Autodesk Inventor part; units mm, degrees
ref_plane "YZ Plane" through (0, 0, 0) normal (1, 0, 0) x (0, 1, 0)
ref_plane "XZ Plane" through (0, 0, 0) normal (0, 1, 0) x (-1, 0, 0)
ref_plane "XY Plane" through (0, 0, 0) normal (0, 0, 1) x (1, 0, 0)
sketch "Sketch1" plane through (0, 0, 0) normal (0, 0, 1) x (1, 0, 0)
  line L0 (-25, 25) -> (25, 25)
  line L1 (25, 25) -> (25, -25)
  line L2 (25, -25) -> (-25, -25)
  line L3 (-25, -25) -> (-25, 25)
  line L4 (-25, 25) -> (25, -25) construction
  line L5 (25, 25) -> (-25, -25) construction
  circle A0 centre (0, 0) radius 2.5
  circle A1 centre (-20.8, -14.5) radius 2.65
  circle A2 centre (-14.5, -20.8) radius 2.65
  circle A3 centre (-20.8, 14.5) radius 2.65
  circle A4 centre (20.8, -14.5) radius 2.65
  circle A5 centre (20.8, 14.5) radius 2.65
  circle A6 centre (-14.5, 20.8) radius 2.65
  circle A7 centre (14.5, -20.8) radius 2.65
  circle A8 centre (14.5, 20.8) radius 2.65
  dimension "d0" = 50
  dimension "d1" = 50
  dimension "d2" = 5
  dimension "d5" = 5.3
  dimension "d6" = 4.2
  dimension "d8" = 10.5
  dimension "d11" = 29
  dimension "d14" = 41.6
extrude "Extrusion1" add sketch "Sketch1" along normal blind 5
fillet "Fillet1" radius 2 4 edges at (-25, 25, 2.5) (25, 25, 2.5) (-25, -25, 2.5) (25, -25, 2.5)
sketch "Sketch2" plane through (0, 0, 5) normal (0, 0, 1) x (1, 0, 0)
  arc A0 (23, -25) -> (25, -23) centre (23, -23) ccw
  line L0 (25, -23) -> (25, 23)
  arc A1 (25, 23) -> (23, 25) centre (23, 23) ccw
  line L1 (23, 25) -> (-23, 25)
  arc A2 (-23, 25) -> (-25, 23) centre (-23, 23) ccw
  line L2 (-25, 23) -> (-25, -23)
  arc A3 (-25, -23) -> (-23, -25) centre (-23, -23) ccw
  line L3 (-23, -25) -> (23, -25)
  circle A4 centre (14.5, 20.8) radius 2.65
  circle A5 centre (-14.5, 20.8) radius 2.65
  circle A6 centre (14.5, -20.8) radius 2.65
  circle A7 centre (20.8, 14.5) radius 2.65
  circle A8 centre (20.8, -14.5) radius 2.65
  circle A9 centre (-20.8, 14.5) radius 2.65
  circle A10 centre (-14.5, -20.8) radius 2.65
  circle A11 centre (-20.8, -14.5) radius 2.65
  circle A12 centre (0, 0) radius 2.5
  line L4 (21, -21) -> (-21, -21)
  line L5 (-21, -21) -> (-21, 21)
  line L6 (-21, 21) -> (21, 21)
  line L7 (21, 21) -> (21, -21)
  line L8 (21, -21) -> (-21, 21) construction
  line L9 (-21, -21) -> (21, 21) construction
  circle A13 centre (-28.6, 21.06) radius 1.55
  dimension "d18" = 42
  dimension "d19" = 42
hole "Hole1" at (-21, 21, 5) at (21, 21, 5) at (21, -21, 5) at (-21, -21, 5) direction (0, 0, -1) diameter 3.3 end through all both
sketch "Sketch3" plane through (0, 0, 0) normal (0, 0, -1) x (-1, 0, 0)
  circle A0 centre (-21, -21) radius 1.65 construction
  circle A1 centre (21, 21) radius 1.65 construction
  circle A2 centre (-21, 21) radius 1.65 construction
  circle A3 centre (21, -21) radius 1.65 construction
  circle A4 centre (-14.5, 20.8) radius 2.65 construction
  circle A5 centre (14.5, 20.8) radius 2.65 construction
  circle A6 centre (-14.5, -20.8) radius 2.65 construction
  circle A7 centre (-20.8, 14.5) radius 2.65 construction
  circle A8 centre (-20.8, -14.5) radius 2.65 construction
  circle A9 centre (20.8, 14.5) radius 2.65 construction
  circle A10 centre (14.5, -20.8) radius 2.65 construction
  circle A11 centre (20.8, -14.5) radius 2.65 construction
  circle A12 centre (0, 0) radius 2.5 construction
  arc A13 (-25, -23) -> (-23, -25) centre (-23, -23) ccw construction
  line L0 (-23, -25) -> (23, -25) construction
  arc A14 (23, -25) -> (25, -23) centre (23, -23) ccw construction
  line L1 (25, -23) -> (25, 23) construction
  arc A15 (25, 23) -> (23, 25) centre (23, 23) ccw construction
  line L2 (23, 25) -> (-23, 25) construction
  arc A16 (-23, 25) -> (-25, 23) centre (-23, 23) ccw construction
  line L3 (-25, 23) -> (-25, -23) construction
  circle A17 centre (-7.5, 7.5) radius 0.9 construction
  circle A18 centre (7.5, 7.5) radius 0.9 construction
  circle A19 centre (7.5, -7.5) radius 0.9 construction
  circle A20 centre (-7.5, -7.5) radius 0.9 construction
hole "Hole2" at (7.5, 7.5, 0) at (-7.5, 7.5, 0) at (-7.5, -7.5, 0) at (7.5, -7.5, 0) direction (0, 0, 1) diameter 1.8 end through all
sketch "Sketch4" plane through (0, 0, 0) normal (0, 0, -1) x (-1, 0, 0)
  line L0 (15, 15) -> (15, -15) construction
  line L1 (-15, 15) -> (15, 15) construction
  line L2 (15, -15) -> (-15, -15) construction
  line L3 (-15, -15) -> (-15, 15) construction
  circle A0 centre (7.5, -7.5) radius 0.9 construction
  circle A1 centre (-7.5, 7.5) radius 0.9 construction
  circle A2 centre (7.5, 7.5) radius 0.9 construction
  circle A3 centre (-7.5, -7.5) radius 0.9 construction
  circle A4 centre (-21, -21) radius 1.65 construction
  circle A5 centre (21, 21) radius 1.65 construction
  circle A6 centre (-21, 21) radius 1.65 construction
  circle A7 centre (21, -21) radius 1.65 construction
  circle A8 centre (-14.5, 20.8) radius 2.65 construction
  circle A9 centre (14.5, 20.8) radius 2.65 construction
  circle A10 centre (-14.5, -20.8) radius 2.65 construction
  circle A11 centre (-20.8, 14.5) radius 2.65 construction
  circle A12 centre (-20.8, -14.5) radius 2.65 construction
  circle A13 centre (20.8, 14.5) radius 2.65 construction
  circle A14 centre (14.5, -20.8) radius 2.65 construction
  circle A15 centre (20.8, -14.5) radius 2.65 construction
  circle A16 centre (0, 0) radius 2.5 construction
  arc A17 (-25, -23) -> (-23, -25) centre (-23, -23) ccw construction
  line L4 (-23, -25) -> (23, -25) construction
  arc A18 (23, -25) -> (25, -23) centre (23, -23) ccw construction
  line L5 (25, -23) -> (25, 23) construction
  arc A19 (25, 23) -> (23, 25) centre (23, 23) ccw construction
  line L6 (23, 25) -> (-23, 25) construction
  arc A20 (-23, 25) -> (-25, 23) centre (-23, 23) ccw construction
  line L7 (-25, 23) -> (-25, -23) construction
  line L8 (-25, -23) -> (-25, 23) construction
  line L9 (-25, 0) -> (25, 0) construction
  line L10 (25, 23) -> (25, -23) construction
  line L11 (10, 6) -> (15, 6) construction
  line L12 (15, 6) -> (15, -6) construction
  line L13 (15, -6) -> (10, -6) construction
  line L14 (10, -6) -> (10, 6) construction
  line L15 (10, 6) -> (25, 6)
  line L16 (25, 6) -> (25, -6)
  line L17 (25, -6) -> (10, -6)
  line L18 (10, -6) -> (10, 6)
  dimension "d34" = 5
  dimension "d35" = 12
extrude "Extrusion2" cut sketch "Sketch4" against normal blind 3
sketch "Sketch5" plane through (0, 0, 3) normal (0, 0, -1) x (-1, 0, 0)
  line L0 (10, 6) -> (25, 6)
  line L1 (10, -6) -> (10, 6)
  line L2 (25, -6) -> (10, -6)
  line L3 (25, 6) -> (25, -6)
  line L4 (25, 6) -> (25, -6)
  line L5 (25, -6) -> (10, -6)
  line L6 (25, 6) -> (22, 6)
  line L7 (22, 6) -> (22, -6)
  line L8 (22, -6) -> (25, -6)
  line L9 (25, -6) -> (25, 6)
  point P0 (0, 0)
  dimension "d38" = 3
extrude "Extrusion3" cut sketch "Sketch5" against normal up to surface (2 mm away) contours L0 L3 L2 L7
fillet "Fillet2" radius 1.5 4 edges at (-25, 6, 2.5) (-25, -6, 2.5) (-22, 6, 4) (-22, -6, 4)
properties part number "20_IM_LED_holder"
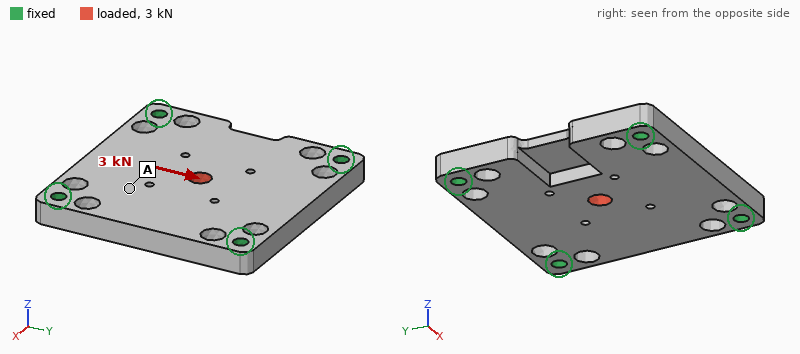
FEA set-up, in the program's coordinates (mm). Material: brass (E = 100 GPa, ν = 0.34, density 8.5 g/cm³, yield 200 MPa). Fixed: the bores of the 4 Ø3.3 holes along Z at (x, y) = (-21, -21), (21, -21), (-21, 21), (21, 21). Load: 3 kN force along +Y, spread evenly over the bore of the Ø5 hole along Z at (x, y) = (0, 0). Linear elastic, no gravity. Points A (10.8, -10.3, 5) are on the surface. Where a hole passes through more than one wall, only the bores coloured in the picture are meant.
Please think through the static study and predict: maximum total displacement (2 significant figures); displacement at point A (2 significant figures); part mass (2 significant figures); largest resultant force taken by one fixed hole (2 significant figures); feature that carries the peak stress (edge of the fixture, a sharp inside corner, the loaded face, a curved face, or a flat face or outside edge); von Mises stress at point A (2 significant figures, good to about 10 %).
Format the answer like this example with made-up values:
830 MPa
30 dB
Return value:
8.1 µm
4.2 µm
91 g
900 N
the loaded face
15 MPa
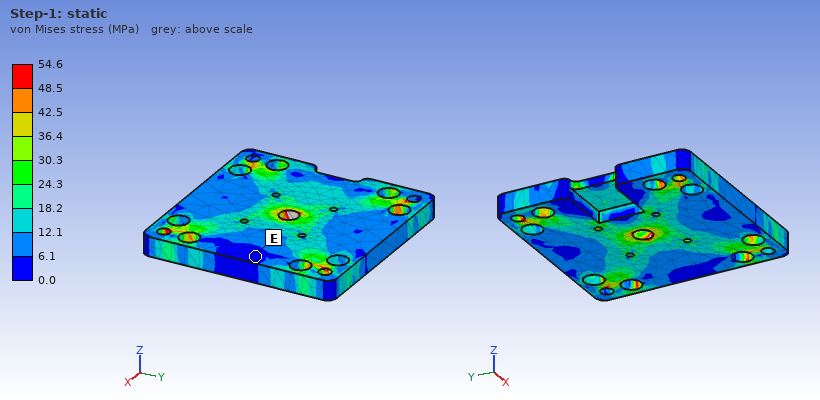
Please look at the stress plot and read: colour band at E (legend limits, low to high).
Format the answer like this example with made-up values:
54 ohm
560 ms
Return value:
0.0 to 6.1 MPa
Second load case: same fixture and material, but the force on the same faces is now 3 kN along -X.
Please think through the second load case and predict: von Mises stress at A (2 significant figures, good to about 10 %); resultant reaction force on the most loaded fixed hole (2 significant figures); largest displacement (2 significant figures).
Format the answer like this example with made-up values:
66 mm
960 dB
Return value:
15 MPa
870 N
8.4 µm
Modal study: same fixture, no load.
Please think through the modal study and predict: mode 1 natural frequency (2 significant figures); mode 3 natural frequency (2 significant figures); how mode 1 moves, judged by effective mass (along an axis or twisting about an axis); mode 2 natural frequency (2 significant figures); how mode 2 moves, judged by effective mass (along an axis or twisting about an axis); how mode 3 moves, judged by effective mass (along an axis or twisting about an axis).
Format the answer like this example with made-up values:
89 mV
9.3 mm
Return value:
5400 Hz
9400 Hz
along Z
9000 Hz
twisting about X
twisting about Y
